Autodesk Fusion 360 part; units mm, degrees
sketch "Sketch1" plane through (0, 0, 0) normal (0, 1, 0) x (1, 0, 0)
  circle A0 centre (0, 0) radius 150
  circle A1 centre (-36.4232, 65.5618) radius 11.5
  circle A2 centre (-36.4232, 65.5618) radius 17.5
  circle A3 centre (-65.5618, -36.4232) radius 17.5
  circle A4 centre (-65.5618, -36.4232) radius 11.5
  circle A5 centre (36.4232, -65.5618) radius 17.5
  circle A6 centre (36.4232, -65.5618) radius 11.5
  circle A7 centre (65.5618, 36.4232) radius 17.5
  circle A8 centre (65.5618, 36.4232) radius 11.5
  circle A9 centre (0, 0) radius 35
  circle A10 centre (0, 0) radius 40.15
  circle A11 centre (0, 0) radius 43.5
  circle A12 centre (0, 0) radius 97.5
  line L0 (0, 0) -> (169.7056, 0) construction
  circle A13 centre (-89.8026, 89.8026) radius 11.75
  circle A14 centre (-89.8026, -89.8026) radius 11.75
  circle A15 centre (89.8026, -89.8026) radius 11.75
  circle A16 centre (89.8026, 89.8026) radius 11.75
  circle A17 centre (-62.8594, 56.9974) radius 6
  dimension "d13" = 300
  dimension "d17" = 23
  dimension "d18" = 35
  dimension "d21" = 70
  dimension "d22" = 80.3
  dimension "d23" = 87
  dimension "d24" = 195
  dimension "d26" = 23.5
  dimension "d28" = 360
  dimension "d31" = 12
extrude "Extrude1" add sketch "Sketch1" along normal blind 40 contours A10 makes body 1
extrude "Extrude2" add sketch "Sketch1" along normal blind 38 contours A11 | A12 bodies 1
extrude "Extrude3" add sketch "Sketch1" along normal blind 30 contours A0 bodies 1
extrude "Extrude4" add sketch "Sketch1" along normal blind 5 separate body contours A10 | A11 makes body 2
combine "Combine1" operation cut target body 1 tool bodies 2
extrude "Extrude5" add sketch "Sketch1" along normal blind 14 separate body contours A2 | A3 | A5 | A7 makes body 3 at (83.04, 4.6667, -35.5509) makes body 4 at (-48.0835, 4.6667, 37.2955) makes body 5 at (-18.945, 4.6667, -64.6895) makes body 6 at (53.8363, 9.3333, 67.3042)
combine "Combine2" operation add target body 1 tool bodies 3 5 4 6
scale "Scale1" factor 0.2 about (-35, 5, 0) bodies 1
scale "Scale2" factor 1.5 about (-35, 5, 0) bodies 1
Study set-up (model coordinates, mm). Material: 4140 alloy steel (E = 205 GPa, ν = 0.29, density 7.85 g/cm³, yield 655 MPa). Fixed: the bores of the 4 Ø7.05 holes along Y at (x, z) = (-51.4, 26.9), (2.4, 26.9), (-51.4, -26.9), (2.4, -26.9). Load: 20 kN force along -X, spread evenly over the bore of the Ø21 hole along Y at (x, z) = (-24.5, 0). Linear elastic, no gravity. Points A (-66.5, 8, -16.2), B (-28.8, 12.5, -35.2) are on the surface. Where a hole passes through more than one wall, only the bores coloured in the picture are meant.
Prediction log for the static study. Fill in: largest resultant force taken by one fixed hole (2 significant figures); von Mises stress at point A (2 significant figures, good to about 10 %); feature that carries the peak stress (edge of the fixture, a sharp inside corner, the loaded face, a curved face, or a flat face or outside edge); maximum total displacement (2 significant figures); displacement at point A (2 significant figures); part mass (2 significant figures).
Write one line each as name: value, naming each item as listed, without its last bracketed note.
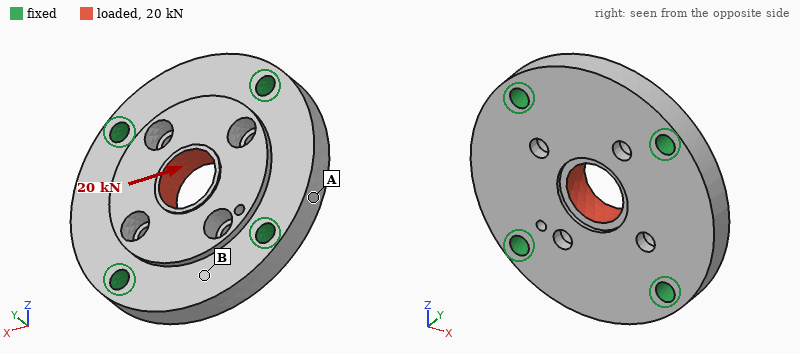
largest resultant force taken by one fixed hole: 5.5 kN
von Mises stress at point A: 19 MPa
feature that carries the peak stress: a curved face
maximum total displacement: 7.7 µm
displacement at point A: 2.9 µm
part mass: 430 g
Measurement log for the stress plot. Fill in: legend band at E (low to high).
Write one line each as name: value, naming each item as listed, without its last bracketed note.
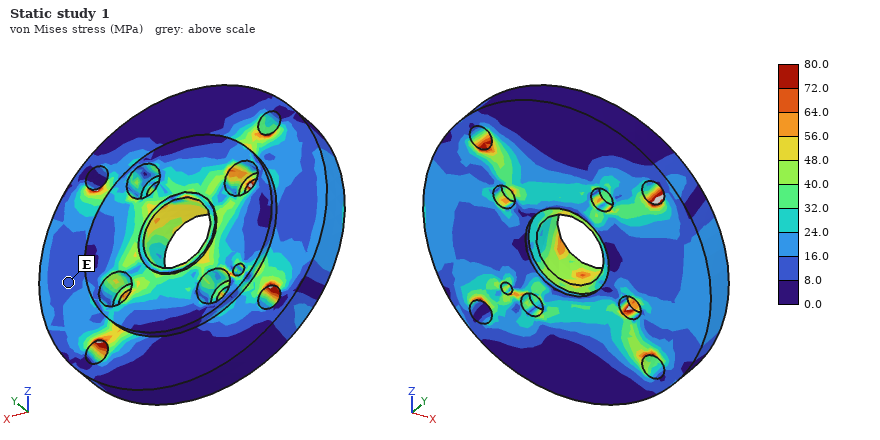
legend band at E: 8.0 to 16.0 MPa
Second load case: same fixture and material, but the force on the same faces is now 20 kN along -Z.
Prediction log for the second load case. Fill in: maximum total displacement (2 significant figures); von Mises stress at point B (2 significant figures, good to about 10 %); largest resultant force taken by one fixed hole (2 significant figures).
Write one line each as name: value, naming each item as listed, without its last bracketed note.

maximum total displacement: 7.6 µm
von Mises stress at point B: 14 MPa
largest resultant force taken by one fixed hole: 5.5 kN
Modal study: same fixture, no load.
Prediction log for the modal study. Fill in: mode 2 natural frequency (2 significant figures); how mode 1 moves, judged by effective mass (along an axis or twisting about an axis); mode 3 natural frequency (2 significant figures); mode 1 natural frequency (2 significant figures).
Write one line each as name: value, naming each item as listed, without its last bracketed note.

mode 2 natural frequency: 12 kHz
how mode 1 moves, judged by effective mass: along Y
mode 3 natural frequency: 13 kHz
mode 1 natural frequency: 12 kHz
